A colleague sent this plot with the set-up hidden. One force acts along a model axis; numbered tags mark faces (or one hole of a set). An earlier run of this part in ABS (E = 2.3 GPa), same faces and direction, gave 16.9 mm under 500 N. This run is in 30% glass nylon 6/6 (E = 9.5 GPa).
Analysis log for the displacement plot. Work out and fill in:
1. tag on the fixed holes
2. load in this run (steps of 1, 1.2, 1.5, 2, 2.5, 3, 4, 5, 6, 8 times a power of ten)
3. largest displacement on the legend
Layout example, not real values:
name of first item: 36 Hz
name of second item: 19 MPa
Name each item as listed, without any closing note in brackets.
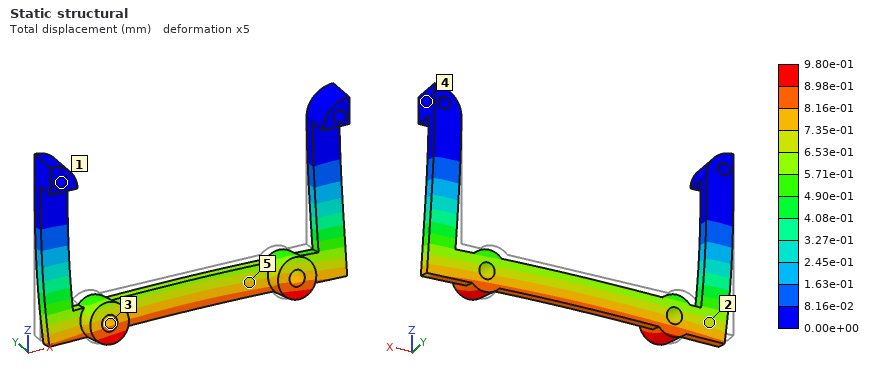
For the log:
tag on the fixed holes: 1
load in this run: 120 N
largest displacement on the legend: 9.80e-01 mm
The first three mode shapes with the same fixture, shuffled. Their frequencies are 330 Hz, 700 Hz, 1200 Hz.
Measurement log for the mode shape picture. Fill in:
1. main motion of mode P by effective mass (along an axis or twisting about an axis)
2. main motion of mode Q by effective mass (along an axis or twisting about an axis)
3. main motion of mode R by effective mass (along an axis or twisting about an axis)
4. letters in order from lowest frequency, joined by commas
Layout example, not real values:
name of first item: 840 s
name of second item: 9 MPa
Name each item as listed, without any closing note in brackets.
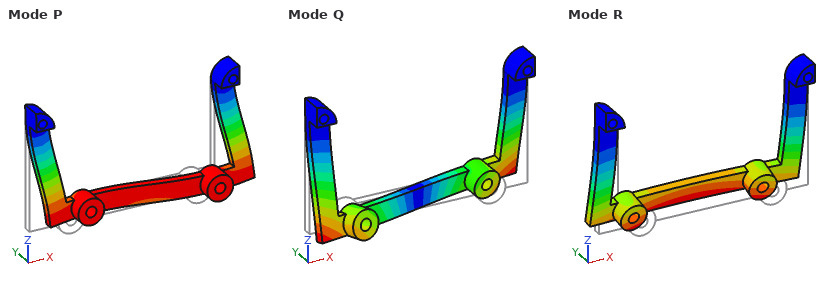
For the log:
main motion of mode P by effective mass: along X
main motion of mode Q by effective mass: twisting about Z
main motion of mode R by effective mass: along Y
letters in order from lowest frequency, joined by commas: R, Q, P
